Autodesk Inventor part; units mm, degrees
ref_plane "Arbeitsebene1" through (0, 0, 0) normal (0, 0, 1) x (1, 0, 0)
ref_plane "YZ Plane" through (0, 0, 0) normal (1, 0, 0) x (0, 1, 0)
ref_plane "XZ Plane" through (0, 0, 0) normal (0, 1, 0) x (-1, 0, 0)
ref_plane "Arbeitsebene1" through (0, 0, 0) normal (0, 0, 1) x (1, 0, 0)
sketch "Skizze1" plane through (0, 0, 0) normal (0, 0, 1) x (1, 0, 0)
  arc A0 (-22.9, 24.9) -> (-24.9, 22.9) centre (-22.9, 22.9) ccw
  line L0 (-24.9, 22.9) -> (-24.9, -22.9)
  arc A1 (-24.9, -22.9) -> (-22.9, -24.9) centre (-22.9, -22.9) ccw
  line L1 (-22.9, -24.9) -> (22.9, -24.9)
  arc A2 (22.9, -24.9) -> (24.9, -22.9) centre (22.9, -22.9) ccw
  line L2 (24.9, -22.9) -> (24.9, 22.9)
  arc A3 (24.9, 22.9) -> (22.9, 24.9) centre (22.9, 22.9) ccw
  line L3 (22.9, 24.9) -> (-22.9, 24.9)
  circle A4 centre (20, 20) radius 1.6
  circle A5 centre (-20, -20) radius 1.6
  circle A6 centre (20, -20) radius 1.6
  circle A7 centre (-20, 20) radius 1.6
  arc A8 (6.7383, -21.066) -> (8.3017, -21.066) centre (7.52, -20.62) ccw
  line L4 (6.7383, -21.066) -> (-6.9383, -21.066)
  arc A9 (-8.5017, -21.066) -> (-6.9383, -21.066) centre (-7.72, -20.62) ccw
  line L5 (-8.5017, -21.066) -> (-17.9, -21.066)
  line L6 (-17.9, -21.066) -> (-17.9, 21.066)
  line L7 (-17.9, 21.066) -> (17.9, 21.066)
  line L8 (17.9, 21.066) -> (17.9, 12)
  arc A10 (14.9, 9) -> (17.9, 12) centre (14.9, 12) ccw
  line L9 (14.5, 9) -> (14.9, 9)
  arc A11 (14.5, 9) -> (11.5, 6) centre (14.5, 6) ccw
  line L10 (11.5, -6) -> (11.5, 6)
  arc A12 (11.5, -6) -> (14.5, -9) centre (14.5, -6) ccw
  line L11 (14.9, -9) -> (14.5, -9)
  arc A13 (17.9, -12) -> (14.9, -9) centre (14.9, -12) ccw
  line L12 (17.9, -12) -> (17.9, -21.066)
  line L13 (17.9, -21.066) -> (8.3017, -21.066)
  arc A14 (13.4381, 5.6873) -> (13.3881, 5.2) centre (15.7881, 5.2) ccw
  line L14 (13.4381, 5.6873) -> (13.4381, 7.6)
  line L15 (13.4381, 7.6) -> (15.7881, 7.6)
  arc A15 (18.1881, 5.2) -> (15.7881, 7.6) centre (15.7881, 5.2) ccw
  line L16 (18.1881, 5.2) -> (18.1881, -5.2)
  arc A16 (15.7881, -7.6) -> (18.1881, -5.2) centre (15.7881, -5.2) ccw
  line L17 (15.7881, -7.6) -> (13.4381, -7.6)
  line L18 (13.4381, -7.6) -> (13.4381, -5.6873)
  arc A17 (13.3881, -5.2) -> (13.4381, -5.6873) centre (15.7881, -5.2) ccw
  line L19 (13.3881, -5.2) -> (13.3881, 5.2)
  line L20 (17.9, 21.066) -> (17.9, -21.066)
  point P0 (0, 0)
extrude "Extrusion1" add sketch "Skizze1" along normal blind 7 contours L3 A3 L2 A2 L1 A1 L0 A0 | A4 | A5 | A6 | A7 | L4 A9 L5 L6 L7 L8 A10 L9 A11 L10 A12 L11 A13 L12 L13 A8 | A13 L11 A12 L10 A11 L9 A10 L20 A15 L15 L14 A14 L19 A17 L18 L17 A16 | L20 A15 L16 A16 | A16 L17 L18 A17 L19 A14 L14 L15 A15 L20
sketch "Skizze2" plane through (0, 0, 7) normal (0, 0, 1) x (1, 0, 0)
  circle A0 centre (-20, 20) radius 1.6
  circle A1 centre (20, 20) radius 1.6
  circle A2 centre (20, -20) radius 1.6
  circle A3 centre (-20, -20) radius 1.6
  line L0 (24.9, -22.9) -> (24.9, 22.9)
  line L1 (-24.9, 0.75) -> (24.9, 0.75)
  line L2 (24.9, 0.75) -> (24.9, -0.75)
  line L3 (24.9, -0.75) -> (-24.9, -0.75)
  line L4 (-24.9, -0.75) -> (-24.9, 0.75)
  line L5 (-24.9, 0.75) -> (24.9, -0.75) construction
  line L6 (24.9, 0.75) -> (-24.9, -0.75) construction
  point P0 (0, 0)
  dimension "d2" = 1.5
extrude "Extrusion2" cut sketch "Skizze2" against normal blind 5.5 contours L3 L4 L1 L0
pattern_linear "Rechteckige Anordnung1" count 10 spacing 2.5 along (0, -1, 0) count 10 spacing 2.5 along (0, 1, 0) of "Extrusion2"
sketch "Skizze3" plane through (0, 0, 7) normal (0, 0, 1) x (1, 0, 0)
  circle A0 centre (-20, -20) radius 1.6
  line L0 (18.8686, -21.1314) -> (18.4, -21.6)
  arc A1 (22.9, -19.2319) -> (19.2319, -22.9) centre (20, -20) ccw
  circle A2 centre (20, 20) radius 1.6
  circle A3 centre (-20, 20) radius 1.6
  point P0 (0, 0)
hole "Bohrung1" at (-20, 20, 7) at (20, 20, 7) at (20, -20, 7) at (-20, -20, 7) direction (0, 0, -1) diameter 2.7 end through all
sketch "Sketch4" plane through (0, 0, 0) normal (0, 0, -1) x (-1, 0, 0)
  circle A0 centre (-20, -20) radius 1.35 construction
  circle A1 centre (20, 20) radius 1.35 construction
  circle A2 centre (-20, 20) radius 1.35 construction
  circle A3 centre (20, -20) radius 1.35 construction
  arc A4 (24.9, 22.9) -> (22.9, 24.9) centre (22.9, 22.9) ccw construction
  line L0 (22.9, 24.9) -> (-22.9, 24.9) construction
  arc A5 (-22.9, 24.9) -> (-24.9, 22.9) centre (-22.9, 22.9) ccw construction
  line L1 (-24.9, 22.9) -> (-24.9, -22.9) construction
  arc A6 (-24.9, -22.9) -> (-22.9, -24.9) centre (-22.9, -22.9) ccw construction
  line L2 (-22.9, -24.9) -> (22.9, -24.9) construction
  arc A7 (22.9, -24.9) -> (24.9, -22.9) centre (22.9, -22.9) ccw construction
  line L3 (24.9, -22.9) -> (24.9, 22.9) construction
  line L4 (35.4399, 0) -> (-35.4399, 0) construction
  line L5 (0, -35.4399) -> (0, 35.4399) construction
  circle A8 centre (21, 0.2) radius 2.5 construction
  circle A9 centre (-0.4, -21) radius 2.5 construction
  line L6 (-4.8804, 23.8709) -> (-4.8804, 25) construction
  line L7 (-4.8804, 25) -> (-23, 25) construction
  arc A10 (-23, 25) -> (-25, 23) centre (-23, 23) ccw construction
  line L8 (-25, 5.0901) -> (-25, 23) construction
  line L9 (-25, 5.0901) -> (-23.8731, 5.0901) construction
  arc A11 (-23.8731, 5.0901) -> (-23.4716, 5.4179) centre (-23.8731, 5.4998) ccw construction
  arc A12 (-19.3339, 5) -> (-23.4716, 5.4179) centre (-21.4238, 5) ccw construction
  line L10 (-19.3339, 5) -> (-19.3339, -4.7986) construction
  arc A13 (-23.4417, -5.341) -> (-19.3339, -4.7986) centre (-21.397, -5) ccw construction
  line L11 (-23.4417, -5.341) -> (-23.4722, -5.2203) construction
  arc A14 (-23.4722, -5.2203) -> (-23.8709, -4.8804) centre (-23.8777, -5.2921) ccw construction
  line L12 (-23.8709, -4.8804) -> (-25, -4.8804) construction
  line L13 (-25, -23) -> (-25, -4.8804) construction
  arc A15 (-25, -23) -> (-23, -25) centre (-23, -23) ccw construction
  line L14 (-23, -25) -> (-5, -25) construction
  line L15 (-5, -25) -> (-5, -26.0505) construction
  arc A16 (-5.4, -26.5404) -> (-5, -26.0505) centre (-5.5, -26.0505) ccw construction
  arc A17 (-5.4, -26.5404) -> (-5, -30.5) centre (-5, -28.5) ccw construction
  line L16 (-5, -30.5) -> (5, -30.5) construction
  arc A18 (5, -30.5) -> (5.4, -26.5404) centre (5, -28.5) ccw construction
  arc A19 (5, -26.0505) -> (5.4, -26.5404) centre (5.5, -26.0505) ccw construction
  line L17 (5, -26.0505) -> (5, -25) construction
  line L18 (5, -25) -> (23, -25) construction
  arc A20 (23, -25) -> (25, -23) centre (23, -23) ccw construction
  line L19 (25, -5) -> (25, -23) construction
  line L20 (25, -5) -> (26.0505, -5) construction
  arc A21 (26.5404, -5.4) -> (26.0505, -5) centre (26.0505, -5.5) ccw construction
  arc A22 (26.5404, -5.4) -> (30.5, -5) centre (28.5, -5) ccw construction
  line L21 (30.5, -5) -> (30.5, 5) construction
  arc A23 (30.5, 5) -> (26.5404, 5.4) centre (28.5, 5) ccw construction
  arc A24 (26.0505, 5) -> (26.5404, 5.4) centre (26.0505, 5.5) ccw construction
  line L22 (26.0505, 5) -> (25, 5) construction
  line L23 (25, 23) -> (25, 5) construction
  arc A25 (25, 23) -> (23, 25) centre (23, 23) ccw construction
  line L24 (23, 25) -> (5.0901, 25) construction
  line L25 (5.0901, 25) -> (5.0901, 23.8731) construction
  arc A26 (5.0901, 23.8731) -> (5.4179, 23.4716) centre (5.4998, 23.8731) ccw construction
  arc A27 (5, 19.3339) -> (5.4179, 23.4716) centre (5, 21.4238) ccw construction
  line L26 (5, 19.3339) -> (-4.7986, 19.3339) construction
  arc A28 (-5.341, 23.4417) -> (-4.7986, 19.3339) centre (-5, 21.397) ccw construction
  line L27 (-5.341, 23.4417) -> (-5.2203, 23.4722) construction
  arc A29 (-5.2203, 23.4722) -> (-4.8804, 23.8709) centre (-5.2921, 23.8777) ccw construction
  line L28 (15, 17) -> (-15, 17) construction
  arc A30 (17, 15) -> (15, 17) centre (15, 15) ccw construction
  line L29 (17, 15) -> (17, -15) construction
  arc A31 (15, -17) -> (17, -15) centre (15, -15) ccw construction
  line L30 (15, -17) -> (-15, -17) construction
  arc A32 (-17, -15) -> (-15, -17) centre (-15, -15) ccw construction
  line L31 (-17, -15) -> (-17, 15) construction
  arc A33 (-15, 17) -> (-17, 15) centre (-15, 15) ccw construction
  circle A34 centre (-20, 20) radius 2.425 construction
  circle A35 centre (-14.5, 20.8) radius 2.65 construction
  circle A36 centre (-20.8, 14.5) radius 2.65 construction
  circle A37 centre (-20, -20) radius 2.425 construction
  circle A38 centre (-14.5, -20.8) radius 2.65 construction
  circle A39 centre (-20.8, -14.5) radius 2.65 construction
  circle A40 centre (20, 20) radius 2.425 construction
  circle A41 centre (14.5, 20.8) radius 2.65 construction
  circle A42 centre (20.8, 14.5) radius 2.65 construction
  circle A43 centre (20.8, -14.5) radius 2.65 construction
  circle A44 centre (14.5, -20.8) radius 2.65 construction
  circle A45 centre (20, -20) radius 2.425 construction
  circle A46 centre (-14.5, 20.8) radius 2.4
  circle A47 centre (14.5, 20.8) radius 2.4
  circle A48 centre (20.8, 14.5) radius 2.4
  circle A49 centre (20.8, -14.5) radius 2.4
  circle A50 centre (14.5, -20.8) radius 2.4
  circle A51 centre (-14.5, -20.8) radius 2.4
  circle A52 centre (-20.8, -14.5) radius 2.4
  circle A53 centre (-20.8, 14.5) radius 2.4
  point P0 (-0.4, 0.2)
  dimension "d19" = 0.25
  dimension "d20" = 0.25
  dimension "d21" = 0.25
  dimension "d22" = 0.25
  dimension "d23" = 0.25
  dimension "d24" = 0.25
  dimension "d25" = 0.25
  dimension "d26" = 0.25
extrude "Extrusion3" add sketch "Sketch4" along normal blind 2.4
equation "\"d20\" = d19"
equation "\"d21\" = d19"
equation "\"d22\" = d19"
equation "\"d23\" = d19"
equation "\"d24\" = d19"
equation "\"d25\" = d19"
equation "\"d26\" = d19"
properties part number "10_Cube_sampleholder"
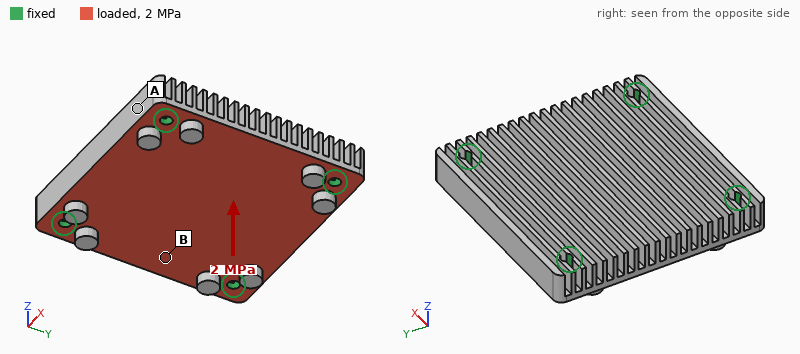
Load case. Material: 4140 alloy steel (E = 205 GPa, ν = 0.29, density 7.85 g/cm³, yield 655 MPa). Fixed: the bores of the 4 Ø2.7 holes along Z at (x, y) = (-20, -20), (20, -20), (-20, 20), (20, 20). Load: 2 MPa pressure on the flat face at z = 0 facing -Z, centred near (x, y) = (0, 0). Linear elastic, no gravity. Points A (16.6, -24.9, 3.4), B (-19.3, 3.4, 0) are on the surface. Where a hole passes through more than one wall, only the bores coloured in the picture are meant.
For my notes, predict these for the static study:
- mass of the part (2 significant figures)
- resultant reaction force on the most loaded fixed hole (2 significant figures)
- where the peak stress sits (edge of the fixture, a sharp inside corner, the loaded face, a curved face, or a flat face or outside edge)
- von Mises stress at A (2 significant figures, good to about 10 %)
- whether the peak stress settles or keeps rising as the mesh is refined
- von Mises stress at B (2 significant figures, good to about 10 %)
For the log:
77 g
1.2 kN
edge of the fixture
59 MPa
keeps rising
240 MPa
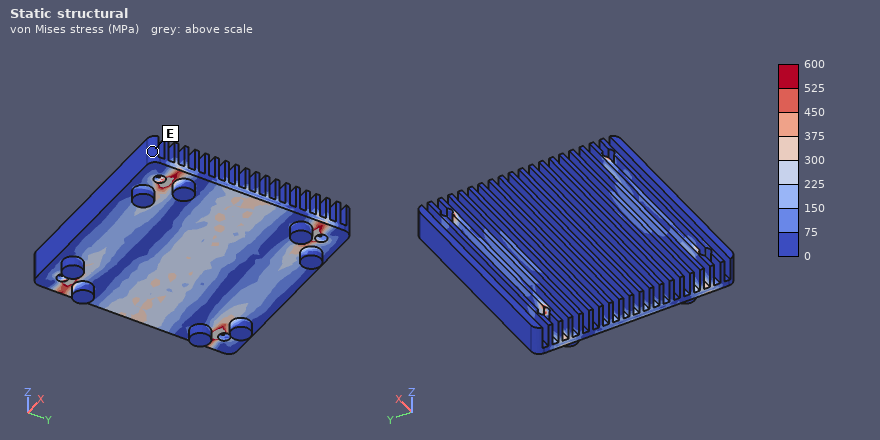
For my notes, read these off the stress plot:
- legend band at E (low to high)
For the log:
0 to 75 MPa
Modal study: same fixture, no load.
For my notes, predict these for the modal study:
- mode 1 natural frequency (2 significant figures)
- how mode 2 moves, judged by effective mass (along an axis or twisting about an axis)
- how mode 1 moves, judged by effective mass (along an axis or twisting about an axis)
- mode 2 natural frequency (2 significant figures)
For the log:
3200 Hz
twisting about Y
along Z
4200 Hz
